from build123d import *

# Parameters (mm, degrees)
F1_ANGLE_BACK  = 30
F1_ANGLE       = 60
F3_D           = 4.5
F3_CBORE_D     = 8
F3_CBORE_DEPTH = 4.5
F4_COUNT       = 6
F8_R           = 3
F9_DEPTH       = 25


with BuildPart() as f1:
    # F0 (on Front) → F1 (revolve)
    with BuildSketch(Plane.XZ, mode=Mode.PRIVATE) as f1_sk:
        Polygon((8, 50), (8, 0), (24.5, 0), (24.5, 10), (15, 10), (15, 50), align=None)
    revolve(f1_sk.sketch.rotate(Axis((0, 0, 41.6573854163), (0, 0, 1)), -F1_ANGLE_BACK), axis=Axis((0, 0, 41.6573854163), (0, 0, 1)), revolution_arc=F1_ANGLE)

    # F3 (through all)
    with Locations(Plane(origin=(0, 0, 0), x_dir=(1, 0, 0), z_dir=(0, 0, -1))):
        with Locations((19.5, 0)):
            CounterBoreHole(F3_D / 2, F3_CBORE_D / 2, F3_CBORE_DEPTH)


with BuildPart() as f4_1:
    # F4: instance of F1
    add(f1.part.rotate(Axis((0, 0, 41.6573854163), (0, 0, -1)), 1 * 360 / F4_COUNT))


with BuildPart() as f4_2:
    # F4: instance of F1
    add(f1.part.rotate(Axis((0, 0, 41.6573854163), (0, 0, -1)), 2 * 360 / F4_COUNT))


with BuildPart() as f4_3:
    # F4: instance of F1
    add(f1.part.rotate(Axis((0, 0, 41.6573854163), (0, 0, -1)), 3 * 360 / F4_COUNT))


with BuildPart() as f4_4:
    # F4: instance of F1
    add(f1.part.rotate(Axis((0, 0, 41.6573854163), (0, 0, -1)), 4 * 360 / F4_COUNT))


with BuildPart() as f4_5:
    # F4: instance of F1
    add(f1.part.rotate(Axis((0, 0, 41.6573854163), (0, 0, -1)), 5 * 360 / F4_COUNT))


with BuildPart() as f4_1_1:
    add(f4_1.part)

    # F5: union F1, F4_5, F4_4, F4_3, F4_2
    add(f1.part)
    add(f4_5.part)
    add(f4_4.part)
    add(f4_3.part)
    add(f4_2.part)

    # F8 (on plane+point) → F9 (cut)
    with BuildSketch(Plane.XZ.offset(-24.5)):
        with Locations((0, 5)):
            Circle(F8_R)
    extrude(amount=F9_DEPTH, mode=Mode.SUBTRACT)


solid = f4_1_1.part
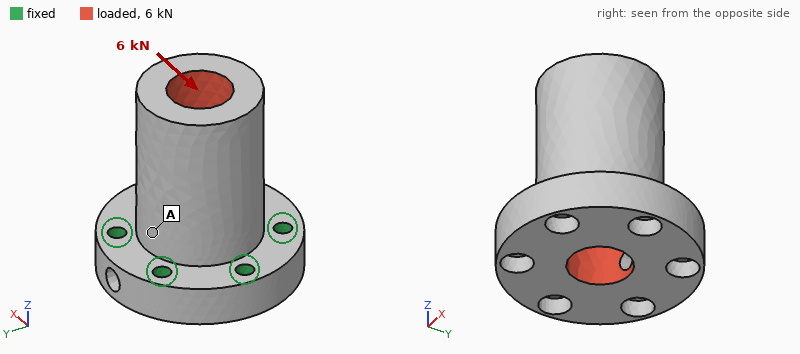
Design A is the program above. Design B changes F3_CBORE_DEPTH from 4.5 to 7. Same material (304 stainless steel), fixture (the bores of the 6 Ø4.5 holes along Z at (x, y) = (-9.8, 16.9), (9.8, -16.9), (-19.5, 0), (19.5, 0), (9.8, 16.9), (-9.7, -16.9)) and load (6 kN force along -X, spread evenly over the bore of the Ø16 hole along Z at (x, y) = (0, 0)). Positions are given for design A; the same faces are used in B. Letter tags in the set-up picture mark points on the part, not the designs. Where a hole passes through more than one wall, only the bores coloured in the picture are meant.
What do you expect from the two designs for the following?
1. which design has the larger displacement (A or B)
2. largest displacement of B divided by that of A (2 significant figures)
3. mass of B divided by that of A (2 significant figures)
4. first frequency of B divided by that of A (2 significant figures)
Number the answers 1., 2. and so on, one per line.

1. B
2. 1.2
3. 0.99
4. 0.92
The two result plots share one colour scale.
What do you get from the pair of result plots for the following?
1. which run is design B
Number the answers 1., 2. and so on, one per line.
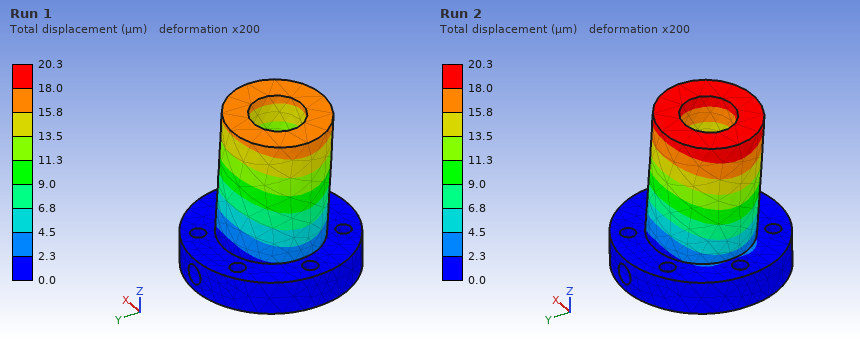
1. Run 2
